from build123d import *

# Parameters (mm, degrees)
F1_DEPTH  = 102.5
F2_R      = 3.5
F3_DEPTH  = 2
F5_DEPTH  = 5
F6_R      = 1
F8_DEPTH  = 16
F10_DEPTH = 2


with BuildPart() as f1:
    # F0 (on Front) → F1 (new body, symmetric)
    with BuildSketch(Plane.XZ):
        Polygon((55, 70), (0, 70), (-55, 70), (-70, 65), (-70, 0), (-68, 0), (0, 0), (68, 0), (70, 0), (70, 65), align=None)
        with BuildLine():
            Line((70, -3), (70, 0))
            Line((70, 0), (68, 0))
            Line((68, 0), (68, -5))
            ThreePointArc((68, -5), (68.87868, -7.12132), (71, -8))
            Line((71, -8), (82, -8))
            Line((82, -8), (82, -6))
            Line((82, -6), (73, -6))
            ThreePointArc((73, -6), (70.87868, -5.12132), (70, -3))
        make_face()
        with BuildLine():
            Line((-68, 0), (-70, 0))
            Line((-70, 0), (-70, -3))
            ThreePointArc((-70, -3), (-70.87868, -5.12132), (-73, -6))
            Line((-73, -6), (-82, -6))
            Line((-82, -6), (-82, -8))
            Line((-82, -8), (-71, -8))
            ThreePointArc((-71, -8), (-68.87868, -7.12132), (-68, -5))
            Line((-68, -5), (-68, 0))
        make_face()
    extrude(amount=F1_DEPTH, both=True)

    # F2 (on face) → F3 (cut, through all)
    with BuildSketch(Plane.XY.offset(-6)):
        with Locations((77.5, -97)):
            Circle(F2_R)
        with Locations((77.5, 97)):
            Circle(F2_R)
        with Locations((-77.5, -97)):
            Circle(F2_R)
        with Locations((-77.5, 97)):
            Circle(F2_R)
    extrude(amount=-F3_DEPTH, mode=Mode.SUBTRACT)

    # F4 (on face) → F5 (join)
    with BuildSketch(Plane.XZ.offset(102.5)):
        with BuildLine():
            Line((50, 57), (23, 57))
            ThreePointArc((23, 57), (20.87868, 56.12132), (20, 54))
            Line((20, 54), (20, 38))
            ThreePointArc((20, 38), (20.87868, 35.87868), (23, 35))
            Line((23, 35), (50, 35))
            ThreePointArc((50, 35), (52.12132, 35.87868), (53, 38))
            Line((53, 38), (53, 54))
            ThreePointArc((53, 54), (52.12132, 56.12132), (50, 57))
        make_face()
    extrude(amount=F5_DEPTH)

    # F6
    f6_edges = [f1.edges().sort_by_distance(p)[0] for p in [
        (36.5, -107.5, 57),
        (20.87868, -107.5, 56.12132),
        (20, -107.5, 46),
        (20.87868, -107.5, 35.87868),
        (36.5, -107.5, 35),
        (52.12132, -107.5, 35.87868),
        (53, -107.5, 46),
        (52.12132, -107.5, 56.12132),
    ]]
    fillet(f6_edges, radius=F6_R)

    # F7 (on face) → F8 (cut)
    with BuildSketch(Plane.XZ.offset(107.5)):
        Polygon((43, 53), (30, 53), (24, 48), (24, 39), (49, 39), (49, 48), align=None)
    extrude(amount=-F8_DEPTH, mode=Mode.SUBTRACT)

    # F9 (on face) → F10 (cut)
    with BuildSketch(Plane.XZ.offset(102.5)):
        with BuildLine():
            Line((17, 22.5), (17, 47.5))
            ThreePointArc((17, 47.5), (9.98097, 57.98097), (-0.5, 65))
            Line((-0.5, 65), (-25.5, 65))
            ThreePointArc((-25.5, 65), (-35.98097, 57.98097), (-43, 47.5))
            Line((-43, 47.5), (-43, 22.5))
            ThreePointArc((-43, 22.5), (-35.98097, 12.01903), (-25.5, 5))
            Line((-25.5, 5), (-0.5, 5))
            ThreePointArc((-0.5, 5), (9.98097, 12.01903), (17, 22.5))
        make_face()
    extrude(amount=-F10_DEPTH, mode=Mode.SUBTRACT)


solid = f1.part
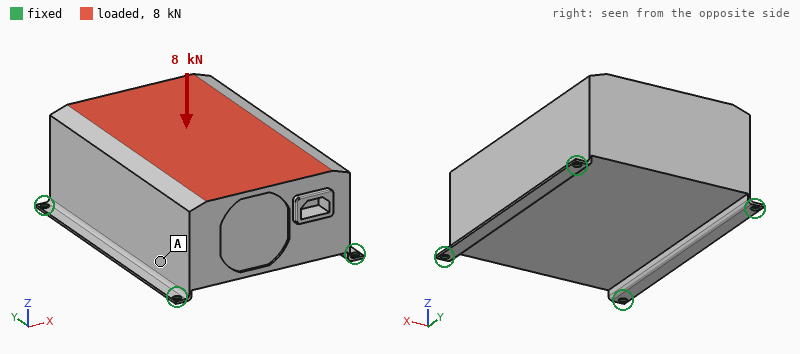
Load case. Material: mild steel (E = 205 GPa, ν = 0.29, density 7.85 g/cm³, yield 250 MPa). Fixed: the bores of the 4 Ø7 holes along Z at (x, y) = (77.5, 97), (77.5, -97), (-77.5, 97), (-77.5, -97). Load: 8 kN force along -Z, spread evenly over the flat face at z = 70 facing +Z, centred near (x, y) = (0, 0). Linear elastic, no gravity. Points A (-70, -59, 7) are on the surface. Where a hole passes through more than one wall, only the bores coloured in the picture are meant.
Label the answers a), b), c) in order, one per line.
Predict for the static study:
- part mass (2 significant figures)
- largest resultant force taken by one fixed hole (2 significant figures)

a) 16 kg
b) 2.4 kN
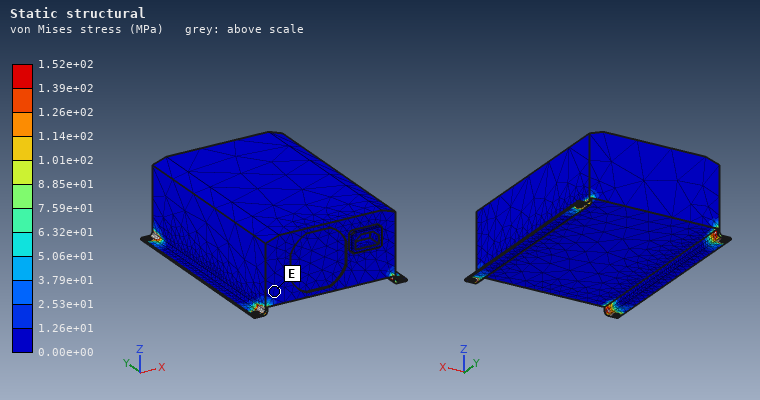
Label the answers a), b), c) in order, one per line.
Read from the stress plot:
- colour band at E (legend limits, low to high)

a) 0.00e+00 to 1.26e+01 MPa
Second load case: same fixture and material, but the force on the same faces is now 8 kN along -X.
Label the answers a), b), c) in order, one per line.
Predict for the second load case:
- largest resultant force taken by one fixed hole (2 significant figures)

a) 3.1 kN
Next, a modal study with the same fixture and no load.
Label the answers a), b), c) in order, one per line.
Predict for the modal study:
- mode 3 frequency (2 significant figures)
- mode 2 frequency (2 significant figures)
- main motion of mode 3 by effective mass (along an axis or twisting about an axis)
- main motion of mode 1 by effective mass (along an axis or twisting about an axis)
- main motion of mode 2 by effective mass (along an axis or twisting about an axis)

a) 930 Hz
b) 770 Hz
c) along Y
d) along X
e) along Z
